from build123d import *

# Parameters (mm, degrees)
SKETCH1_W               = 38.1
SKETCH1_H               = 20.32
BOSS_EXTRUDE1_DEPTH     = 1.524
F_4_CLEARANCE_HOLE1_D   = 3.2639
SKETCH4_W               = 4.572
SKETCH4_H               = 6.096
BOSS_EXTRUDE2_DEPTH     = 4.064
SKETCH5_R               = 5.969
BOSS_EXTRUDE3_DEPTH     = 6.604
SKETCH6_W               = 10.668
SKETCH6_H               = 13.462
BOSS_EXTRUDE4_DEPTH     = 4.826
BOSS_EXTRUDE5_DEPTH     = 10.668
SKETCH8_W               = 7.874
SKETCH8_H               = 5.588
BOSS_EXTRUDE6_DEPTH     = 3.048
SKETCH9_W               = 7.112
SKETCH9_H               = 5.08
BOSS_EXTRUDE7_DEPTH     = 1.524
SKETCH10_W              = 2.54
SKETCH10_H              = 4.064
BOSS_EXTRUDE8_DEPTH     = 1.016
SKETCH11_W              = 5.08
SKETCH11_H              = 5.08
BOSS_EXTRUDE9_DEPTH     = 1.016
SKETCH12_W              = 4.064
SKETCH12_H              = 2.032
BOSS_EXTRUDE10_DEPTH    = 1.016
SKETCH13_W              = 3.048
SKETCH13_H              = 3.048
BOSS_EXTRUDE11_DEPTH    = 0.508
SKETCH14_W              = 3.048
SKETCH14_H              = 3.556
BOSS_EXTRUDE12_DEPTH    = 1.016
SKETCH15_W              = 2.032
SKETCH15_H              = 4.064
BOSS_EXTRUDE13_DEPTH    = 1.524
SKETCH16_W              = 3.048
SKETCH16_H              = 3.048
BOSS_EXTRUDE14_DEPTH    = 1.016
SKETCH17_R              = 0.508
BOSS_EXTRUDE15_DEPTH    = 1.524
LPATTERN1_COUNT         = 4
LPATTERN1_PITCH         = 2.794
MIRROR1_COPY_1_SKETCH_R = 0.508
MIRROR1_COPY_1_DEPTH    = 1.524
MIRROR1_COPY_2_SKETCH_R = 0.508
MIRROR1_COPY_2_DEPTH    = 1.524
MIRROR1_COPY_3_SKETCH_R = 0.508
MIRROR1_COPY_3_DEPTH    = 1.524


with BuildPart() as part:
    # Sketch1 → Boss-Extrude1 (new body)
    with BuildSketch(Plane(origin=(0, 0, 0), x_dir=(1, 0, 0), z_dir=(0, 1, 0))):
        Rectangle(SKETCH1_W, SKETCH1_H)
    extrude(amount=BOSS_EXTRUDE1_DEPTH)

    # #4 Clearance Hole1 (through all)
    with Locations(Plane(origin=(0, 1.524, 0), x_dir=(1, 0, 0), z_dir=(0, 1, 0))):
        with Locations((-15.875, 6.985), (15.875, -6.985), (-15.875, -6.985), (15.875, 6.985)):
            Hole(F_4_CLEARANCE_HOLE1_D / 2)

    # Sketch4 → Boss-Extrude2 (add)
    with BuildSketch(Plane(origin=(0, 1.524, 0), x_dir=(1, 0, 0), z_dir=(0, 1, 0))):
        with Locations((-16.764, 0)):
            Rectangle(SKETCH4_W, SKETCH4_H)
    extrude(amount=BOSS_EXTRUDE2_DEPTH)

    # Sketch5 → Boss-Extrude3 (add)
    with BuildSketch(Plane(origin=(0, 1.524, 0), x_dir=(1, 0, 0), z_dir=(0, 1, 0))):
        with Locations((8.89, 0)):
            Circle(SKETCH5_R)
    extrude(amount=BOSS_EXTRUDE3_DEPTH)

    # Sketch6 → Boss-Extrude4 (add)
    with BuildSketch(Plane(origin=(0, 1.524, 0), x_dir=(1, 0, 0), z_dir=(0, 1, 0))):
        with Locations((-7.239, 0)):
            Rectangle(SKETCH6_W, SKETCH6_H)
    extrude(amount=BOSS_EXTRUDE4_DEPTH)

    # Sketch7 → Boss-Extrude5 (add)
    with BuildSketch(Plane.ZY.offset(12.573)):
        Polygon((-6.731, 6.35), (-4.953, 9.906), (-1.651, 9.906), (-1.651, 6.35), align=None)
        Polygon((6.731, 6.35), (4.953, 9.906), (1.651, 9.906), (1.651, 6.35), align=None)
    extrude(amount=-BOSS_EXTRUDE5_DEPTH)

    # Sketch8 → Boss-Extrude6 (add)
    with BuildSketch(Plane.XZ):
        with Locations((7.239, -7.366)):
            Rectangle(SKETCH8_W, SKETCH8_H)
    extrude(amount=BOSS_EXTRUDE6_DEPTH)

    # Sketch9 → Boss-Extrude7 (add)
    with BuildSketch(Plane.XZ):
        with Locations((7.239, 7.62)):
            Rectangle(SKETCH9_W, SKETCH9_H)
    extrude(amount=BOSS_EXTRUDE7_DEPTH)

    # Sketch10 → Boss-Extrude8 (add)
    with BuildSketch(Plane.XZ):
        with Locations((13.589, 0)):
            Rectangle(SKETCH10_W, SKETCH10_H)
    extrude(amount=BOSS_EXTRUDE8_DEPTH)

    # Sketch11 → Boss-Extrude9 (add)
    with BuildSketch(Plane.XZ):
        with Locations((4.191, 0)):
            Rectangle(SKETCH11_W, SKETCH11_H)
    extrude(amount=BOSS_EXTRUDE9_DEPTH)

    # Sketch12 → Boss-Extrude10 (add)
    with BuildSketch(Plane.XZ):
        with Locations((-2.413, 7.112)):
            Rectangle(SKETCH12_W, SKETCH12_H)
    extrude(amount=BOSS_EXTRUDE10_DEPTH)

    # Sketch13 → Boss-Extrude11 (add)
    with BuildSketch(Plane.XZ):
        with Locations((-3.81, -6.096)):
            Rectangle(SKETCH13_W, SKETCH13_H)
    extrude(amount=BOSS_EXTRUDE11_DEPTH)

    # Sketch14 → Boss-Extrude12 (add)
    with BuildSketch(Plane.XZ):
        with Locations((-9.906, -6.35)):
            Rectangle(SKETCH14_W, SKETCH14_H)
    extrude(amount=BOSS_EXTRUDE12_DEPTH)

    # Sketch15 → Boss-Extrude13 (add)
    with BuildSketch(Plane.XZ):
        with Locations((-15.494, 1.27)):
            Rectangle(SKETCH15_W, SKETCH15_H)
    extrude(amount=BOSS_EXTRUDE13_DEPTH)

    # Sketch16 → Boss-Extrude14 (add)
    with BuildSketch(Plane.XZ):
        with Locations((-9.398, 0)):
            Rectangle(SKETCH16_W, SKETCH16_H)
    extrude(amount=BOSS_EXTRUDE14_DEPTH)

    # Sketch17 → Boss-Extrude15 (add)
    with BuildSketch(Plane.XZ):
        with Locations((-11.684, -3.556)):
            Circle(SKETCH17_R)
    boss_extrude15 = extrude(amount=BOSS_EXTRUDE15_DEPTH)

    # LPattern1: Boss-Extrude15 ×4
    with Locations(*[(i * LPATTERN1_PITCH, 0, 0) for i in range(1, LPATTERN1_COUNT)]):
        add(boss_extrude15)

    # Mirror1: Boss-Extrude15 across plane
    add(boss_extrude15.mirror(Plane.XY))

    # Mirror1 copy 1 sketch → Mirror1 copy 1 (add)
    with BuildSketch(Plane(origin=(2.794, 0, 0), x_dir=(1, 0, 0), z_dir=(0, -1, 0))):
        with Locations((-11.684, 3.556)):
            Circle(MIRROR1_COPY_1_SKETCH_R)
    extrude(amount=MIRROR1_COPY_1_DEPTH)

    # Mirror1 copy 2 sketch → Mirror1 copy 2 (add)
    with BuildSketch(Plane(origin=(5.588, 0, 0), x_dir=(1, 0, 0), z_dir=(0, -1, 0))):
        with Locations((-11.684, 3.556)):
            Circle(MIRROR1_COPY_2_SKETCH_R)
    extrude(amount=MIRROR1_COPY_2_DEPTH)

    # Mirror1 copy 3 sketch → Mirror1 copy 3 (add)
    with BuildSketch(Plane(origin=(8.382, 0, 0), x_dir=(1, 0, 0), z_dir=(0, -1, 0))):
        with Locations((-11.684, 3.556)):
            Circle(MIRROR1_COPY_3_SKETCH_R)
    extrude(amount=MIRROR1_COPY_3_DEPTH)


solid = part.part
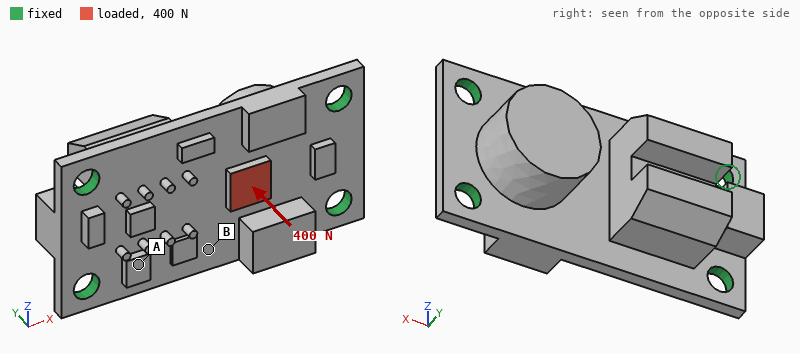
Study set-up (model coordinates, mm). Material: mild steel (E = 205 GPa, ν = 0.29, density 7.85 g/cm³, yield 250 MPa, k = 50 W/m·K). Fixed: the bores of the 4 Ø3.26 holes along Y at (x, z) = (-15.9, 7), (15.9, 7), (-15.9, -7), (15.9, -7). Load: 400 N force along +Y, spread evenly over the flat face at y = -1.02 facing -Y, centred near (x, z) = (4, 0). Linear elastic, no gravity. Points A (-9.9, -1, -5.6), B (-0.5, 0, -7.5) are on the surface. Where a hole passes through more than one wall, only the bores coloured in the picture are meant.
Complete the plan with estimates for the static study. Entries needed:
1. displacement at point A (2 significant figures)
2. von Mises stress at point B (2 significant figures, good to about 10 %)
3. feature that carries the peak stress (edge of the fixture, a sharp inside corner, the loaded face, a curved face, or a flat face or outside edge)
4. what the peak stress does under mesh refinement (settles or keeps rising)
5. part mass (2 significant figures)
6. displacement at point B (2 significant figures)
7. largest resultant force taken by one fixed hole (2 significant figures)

8.7 µm
89 MPa
edge of the fixture
keeps rising
26 g
26 µm
150 N
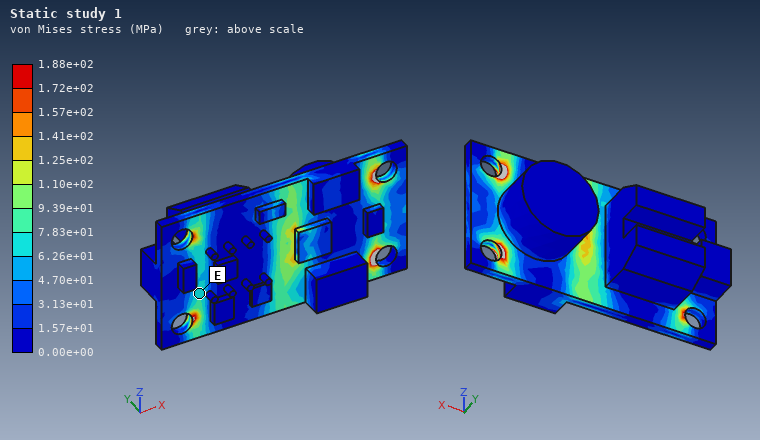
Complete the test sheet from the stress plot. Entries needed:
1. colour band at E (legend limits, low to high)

6.26e+01 to 7.83e+01 MPa
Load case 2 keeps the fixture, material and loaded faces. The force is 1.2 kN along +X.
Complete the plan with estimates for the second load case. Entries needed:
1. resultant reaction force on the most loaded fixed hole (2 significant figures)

380 N
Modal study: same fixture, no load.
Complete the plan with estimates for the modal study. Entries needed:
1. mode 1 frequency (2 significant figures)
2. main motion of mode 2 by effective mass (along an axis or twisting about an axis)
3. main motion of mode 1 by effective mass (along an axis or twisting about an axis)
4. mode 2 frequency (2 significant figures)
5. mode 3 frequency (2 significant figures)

5600 Hz
along Z
along Y
17 kHz
23 kHz
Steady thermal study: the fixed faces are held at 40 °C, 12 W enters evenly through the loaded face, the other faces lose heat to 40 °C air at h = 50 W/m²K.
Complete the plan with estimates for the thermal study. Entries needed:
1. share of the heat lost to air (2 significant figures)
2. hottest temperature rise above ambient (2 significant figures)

16 %
54 K
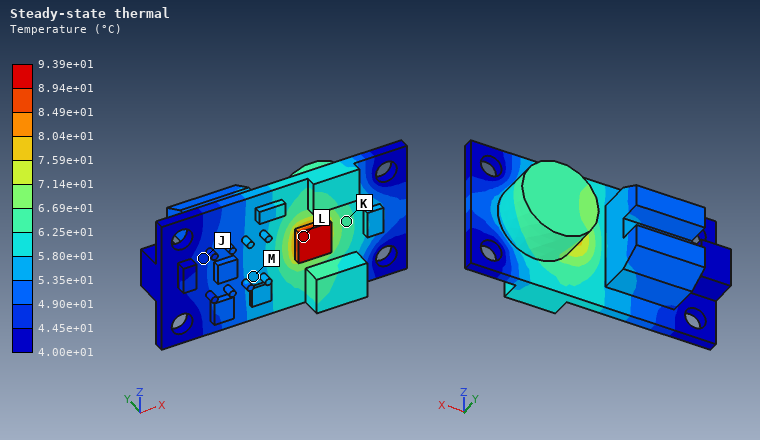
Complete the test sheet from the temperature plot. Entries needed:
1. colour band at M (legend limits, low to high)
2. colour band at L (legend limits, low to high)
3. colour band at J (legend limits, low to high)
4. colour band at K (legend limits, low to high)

5.35e+01 to 5.80e+01 °C
8.94e+01 to 9.39e+01 °C
4.45e+01 to 4.90e+01 °C
6.25e+01 to 6.69e+01 °C
